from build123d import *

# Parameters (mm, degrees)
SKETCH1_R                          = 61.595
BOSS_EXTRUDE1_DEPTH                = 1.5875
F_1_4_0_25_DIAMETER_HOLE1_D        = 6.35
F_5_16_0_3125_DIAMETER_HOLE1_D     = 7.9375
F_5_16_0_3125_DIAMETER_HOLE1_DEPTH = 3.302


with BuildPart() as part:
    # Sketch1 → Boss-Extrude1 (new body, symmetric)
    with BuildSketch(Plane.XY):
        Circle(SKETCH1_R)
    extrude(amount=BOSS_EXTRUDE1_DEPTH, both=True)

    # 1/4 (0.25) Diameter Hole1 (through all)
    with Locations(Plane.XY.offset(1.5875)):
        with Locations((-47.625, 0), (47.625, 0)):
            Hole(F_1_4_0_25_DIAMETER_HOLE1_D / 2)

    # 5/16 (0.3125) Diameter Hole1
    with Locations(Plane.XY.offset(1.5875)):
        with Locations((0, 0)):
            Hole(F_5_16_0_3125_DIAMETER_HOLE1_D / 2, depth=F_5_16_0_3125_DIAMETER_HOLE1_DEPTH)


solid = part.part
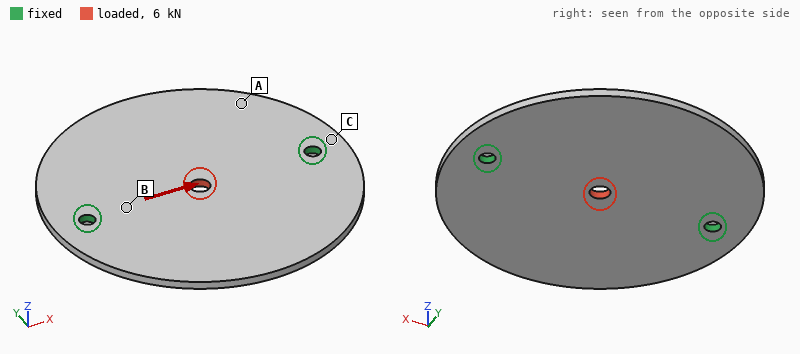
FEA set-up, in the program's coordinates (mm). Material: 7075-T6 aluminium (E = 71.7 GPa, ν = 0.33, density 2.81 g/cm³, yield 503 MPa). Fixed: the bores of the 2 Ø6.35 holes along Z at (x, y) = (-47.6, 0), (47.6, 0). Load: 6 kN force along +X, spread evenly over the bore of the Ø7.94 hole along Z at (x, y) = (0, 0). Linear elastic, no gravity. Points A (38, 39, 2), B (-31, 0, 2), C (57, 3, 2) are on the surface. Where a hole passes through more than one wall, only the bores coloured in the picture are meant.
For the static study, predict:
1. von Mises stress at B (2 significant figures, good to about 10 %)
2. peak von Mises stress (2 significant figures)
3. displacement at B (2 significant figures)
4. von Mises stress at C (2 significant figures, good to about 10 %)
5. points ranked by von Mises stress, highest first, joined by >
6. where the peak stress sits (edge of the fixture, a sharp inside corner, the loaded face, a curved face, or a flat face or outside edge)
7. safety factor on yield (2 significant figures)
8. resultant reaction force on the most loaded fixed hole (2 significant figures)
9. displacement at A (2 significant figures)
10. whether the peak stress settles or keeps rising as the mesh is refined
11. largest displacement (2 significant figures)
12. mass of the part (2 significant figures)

37 MPa
130 MPa
9.1 µm
16 MPa
B > C > A
the loaded face
3.8
3.0 kN
11 µm
settles
26 µm
110 g
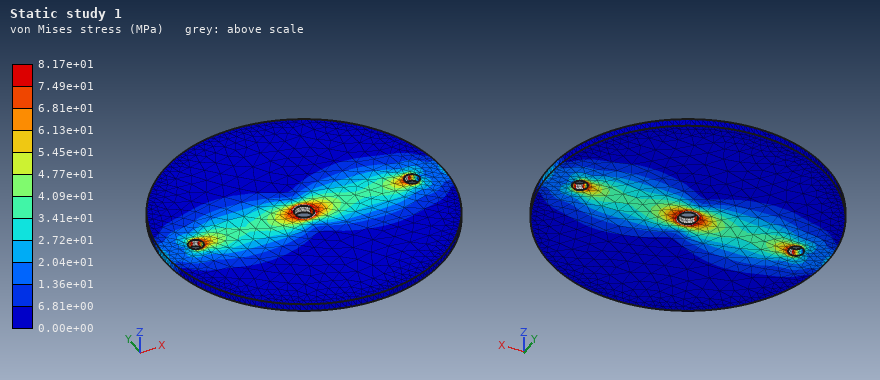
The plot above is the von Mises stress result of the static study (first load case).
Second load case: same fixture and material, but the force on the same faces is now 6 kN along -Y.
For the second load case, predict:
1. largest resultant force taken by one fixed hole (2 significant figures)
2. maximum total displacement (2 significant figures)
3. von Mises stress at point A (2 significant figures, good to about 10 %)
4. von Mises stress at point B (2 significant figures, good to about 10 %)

3.0 kN
34 µm
13 MPa
16 MPa
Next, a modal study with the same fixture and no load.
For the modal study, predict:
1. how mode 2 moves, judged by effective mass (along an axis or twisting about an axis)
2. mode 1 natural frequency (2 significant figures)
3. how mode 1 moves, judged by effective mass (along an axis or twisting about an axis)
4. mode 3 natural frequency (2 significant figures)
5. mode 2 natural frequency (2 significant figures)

along Z
620 Hz
twisting about X
1800 Hz
810 Hz
